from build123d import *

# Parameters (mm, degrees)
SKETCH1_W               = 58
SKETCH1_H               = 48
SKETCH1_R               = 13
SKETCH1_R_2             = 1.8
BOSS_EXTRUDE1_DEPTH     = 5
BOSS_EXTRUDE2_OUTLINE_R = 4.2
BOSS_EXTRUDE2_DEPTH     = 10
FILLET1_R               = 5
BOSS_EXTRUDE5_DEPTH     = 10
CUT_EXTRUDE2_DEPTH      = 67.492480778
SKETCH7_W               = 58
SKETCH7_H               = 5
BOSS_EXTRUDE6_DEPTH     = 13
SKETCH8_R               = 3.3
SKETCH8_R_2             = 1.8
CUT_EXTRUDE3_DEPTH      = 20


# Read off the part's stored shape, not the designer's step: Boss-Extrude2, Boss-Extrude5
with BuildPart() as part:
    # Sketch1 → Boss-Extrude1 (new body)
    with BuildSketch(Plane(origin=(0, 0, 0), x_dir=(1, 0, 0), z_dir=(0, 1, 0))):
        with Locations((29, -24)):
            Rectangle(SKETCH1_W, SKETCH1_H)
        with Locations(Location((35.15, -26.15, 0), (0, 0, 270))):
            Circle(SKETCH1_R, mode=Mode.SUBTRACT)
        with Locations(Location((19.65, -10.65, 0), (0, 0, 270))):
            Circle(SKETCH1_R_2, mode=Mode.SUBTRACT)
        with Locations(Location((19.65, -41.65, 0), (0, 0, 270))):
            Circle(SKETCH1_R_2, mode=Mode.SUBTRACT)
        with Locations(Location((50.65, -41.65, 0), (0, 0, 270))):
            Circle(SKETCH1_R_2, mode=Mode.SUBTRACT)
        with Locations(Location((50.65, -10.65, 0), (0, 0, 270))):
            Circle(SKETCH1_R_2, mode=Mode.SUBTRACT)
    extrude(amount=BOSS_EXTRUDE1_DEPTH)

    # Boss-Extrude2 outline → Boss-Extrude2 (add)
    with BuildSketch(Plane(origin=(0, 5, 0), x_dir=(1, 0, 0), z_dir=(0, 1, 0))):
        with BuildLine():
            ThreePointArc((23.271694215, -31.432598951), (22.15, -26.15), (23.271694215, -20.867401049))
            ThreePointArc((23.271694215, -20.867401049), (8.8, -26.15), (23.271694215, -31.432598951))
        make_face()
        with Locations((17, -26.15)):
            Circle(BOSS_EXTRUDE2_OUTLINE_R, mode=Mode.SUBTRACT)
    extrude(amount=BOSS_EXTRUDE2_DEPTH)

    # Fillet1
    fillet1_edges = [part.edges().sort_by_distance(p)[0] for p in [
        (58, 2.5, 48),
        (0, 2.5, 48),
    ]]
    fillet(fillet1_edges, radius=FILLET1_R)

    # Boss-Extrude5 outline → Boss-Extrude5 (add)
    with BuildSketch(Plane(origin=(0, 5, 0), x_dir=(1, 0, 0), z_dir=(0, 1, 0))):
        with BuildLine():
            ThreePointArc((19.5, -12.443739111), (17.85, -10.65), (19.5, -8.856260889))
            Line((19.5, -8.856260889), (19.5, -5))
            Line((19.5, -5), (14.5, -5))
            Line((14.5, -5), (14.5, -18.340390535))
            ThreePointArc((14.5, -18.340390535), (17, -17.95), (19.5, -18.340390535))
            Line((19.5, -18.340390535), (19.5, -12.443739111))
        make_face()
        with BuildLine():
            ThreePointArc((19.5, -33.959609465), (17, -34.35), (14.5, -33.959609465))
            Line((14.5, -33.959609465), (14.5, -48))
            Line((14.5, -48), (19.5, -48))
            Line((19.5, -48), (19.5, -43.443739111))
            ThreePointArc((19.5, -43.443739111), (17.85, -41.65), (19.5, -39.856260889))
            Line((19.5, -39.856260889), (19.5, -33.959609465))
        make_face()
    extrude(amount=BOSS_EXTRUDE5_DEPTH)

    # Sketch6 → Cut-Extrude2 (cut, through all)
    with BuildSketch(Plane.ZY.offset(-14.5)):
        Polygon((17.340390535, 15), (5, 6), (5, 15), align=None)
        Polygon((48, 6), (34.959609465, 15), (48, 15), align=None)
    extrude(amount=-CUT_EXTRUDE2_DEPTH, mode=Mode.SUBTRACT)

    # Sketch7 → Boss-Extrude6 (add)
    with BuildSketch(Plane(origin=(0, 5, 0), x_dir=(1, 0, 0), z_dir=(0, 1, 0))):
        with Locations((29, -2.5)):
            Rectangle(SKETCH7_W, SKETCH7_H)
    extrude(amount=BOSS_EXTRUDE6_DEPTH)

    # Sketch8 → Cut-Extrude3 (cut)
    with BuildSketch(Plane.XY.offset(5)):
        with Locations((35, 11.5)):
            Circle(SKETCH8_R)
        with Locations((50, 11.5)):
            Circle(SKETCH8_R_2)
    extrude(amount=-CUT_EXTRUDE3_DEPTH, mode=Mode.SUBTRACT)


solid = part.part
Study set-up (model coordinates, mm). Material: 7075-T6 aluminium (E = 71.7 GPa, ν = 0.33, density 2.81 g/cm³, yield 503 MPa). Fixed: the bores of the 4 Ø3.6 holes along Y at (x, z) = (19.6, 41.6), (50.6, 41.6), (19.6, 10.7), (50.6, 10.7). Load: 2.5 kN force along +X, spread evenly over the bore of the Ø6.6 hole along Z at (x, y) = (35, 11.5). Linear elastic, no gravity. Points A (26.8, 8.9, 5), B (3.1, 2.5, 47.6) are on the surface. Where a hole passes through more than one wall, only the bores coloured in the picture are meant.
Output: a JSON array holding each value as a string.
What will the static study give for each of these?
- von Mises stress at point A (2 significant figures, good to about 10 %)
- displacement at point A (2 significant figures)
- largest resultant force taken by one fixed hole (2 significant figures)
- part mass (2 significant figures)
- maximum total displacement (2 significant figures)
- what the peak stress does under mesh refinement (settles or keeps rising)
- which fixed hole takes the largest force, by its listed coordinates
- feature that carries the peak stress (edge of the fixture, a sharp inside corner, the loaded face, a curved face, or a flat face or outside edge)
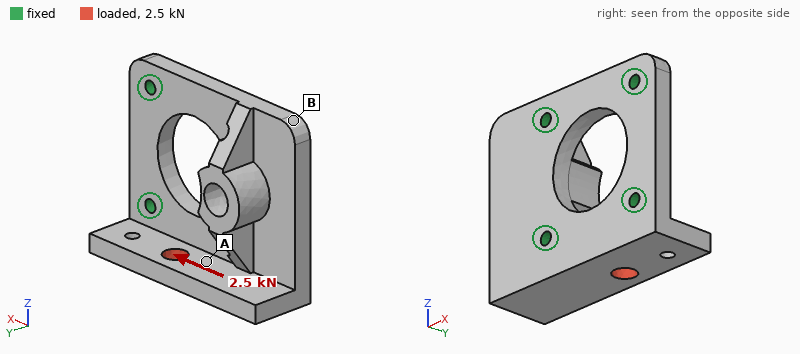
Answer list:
["33 MPa", "9.4 µm", "1.6 kN", "47 g", "27 µm", "keeps rising", "(19.6, 10.7)", "edge of the fixture"]
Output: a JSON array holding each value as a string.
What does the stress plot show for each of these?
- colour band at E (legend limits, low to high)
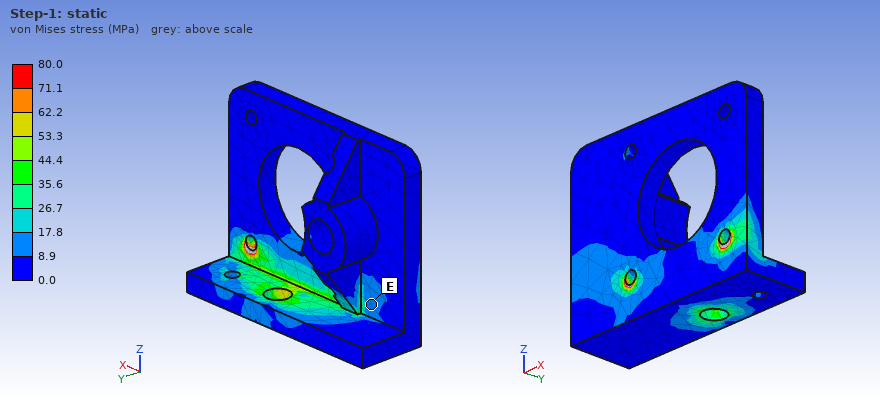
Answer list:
["8.9 to 17.8 MPa"]
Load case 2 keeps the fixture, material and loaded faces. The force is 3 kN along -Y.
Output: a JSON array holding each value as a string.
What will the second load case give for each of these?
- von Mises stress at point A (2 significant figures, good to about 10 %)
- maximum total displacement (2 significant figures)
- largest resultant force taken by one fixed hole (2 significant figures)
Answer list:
["27 MPa", "75 µm", "1.8 kN"]
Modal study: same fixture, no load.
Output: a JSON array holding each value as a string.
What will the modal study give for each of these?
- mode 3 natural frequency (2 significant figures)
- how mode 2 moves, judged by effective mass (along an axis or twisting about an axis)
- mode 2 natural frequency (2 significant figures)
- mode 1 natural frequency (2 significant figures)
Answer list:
["11 kHz", "along Y", "9800 Hz", "8900 Hz"]
